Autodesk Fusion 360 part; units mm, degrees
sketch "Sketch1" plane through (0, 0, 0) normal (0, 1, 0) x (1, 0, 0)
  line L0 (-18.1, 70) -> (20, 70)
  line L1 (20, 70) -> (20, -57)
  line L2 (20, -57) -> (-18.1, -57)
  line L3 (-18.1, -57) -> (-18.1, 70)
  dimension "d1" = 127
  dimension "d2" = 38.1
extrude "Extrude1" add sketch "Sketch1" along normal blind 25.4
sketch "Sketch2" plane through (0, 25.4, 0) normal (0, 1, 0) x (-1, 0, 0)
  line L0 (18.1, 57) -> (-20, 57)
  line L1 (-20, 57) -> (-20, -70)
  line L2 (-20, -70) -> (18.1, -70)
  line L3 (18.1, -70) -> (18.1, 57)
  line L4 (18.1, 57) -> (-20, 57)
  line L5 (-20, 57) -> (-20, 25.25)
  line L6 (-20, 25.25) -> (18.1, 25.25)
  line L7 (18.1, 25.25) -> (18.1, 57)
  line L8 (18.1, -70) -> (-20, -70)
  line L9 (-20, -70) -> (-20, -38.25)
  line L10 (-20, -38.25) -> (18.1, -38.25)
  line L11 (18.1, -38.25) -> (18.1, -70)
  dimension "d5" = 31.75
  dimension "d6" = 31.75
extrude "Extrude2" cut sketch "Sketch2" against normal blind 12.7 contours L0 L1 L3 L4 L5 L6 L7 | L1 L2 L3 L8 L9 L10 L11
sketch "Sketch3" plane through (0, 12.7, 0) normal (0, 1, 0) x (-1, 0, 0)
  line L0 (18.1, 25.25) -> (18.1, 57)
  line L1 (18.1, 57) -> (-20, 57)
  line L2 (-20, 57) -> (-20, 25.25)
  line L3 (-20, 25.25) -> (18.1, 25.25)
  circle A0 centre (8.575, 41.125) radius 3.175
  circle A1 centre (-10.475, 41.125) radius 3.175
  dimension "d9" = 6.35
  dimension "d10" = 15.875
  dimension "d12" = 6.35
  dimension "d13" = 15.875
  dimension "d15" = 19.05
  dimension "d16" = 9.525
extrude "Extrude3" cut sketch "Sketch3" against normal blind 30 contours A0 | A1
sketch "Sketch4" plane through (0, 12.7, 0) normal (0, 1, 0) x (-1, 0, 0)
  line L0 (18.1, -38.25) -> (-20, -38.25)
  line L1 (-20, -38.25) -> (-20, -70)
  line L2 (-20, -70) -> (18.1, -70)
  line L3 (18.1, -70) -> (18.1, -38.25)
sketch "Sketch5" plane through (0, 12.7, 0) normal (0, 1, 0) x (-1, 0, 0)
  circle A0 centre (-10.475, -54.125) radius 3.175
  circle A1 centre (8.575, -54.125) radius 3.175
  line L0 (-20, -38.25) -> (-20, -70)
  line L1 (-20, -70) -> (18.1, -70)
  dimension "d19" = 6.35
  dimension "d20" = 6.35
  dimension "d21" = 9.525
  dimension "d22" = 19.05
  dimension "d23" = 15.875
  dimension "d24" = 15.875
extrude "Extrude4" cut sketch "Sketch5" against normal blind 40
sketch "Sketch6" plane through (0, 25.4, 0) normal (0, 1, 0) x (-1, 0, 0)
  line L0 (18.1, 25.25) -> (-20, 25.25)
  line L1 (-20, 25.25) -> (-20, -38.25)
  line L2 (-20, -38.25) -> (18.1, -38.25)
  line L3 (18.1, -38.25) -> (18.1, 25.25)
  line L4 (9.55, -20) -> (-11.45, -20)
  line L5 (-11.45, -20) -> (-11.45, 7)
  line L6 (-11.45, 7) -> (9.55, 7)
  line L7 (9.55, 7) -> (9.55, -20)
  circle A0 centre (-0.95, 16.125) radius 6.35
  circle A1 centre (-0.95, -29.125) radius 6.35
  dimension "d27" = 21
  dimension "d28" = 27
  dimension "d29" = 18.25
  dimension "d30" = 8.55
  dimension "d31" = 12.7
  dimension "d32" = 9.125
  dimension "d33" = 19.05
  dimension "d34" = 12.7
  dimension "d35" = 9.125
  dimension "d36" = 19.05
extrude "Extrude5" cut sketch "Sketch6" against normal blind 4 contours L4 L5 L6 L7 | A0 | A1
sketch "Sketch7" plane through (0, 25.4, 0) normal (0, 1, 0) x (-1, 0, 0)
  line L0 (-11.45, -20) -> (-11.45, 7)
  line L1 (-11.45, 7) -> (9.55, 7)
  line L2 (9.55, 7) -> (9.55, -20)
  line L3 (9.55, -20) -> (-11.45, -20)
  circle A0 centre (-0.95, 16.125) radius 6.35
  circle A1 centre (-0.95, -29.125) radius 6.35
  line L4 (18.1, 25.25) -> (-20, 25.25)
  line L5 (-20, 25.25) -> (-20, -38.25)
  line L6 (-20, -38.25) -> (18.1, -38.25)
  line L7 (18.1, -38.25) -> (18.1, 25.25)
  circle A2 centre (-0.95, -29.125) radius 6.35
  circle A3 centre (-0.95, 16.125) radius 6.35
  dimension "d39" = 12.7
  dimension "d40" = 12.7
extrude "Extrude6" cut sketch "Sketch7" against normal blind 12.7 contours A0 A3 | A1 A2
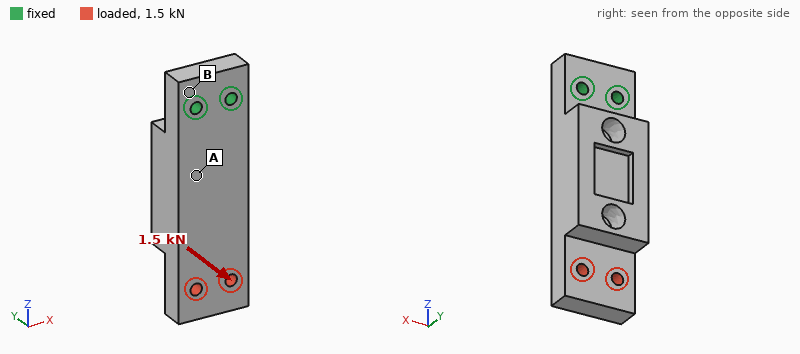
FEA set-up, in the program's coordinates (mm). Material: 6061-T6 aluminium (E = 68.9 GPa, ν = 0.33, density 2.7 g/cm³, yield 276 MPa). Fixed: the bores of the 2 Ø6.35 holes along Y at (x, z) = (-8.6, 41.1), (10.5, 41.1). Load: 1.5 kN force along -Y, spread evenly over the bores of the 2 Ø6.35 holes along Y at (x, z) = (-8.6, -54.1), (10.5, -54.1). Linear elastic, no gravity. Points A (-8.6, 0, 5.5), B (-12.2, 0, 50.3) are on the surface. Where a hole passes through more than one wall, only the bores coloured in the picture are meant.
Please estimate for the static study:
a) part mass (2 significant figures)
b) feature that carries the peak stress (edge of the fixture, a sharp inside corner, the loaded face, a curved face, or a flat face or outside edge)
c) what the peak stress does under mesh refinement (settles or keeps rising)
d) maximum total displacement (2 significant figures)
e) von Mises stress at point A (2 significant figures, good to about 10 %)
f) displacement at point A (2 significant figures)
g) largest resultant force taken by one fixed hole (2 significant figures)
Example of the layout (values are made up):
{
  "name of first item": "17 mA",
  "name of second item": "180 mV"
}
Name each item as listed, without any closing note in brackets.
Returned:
{
  "part mass": "230 g",
  "feature that carries the peak stress": "edge of the fixture",
  "what the peak stress does under mesh refinement": "keeps rising",
  "maximum total displacement": "0.71 mm",
  "von Mises stress at point A": "29 MPa",
  "displacement at point A": "0.16 mm",
  "largest resultant force taken by one fixed hole": "750 N"
}
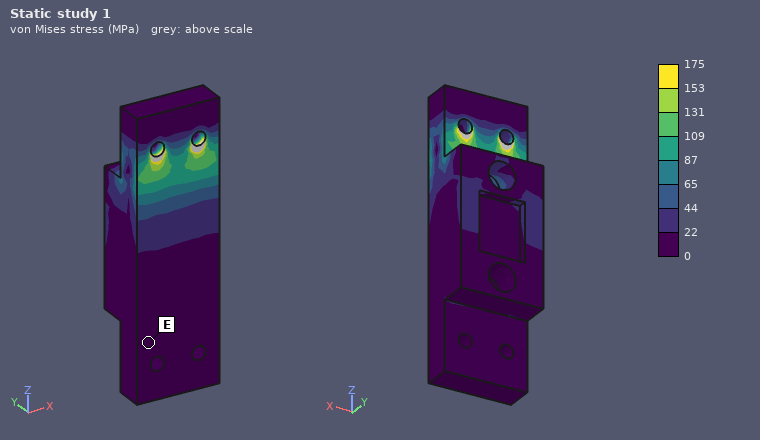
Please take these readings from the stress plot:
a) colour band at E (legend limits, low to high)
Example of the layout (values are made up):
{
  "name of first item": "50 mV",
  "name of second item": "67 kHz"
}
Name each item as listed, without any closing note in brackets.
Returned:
{
  "colour band at E": "0 to 22 MPa"
}
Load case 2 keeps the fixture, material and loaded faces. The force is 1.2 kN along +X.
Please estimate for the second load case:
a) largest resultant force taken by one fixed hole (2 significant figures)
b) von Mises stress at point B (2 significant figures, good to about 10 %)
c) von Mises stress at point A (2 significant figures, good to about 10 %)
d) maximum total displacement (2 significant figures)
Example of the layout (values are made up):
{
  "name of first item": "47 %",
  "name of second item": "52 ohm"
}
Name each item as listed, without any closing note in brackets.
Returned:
{
  "largest resultant force taken by one fixed hole": "5.0 kN",
  "von Mises stress at point B": "5.6 MPa",
  "von Mises stress at point A": "12 MPa",
  "maximum total displacement": "0.11 mm"
}
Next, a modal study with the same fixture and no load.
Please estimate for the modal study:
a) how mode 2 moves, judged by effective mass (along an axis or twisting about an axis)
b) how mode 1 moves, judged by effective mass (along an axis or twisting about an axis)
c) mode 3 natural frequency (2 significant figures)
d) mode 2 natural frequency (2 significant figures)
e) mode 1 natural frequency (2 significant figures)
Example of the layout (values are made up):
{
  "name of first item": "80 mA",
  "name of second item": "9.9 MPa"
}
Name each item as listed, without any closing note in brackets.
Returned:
{
  "how mode 2 moves, judged by effective mass": "along X",
  "how mode 1 moves, judged by effective mass": "along Y",
  "mode 3 natural frequency": "4600 Hz",
  "mode 2 natural frequency": "2200 Hz",
  "mode 1 natural frequency": "940 Hz"
}
